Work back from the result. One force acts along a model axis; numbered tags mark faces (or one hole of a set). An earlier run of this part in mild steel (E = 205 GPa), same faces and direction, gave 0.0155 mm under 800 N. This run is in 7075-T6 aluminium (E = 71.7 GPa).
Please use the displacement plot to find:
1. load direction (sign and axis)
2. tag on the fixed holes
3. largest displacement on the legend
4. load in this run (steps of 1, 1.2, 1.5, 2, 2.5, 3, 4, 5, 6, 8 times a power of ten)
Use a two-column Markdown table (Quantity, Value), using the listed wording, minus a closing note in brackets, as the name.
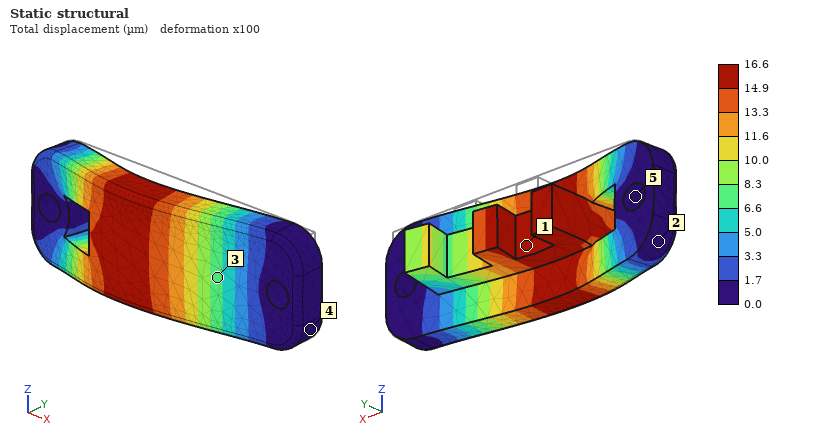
| Quantity | Value |
|---|---|
| load direction | -Y |
| tag on the fixed holes | 5 |
| largest displacement on the legend | 16.6 µm |
| load in this run | 300 N |
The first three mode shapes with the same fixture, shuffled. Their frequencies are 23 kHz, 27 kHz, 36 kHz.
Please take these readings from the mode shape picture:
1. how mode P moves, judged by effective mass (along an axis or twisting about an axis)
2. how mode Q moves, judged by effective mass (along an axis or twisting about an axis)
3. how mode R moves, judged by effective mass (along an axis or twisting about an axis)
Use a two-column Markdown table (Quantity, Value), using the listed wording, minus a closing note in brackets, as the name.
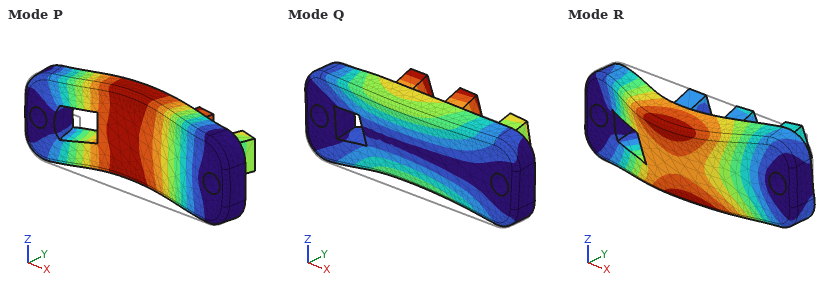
| Quantity | Value |
|---|---|
| how mode P moves, judged by effective mass | along Y |
| how mode Q moves, judged by effective mass | along Z |
| how mode R moves, judged by effective mass | along Z |
